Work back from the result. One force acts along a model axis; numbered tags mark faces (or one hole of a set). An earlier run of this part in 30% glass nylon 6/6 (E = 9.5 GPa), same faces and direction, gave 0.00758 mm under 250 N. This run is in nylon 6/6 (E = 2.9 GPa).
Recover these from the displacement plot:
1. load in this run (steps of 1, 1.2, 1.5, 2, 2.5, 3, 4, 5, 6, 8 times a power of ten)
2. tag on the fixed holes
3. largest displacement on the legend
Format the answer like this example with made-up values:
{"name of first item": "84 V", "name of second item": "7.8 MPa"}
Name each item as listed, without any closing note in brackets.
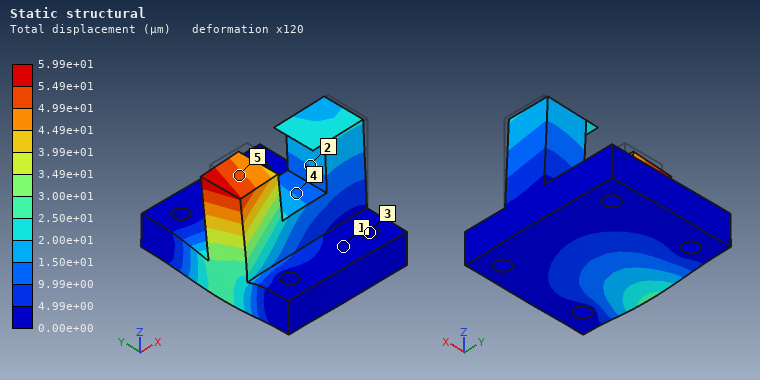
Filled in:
{"load in this run": "600 N", "tag on the fixed holes": "3", "largest displacement on the legend": "5.99e+01 µm"}
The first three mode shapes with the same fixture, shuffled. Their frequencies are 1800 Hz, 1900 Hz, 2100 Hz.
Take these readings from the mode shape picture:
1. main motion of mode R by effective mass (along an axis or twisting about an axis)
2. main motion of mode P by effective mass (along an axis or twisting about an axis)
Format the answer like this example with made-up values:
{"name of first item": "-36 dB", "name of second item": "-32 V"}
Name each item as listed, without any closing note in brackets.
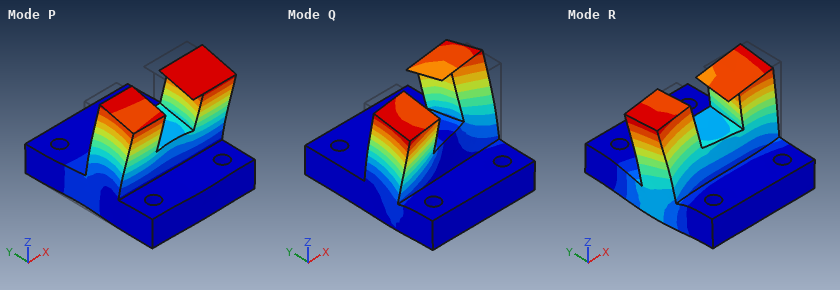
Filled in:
{"main motion of mode R by effective mass": "along X", "main motion of mode P by effective mass": "along Y"}
